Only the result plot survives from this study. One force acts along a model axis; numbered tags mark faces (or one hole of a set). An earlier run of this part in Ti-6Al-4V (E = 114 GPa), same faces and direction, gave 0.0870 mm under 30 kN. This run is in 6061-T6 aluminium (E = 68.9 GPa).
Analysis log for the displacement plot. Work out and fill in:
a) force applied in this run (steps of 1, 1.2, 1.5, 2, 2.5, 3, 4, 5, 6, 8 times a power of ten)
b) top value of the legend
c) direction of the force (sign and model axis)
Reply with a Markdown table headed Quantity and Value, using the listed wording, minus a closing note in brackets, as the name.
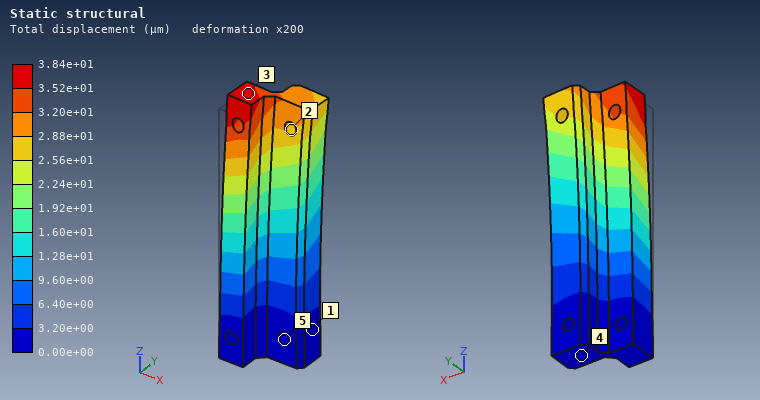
| Quantity | Value |
|---|---|
| force applied in this run | 8 kN |
| top value of the legend | 3.84e+01 µm |
| direction of the force | +Z |
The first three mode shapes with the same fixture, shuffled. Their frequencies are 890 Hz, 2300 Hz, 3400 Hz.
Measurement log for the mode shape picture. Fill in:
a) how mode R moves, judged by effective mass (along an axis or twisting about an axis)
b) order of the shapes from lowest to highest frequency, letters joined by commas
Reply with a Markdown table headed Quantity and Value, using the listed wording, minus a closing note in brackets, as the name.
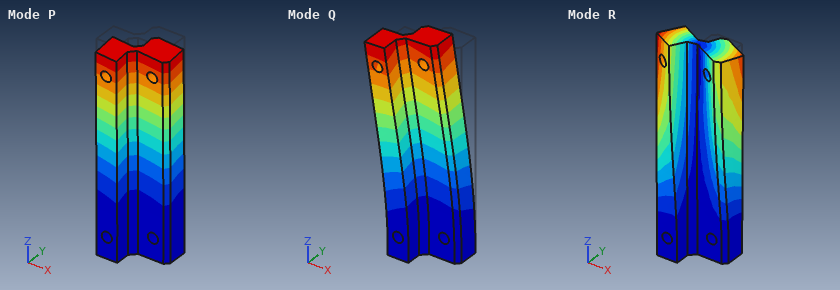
| Quantity | Value |
|---|---|
| how mode R moves, judged by effective mass | twisting about Z |
| order of the shapes from lowest to highest frequency, letters joined by commas | P, Q, R |
